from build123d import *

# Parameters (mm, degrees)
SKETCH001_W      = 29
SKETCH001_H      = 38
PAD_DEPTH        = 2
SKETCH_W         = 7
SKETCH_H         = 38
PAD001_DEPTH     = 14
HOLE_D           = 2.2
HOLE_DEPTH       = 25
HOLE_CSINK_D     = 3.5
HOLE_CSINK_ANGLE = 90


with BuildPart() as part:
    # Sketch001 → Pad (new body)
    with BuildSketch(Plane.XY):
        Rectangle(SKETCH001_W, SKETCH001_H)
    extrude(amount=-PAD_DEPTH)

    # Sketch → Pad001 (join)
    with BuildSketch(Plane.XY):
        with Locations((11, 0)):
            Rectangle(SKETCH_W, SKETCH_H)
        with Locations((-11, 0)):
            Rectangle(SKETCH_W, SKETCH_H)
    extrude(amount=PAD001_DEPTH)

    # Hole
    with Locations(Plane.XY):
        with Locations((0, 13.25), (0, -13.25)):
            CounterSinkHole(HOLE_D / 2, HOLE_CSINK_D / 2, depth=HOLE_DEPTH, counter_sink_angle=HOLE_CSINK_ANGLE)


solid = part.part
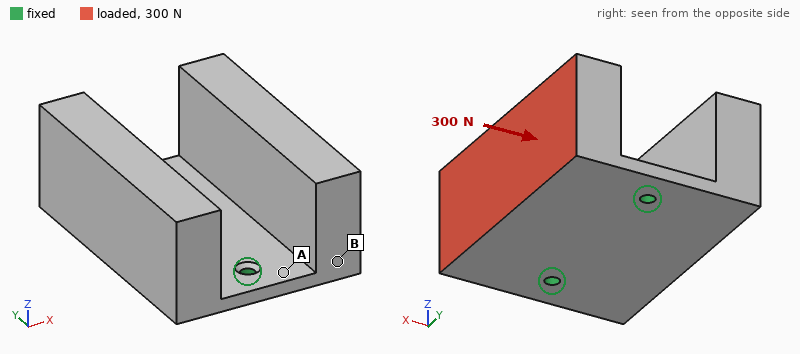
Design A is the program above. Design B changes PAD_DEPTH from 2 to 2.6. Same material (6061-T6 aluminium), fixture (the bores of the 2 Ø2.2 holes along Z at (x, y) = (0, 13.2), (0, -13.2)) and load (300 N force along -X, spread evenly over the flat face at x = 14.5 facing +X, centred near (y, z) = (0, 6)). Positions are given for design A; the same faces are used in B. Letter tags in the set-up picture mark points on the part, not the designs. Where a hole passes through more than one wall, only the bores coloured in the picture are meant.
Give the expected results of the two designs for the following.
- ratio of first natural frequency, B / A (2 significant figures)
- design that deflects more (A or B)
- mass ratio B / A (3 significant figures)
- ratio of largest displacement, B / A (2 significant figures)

1.4
A
1.07
0.48
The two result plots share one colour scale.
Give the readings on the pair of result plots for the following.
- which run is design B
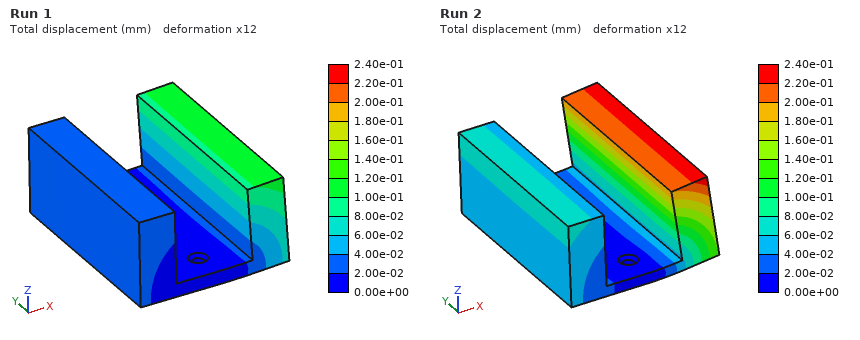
Run 1
